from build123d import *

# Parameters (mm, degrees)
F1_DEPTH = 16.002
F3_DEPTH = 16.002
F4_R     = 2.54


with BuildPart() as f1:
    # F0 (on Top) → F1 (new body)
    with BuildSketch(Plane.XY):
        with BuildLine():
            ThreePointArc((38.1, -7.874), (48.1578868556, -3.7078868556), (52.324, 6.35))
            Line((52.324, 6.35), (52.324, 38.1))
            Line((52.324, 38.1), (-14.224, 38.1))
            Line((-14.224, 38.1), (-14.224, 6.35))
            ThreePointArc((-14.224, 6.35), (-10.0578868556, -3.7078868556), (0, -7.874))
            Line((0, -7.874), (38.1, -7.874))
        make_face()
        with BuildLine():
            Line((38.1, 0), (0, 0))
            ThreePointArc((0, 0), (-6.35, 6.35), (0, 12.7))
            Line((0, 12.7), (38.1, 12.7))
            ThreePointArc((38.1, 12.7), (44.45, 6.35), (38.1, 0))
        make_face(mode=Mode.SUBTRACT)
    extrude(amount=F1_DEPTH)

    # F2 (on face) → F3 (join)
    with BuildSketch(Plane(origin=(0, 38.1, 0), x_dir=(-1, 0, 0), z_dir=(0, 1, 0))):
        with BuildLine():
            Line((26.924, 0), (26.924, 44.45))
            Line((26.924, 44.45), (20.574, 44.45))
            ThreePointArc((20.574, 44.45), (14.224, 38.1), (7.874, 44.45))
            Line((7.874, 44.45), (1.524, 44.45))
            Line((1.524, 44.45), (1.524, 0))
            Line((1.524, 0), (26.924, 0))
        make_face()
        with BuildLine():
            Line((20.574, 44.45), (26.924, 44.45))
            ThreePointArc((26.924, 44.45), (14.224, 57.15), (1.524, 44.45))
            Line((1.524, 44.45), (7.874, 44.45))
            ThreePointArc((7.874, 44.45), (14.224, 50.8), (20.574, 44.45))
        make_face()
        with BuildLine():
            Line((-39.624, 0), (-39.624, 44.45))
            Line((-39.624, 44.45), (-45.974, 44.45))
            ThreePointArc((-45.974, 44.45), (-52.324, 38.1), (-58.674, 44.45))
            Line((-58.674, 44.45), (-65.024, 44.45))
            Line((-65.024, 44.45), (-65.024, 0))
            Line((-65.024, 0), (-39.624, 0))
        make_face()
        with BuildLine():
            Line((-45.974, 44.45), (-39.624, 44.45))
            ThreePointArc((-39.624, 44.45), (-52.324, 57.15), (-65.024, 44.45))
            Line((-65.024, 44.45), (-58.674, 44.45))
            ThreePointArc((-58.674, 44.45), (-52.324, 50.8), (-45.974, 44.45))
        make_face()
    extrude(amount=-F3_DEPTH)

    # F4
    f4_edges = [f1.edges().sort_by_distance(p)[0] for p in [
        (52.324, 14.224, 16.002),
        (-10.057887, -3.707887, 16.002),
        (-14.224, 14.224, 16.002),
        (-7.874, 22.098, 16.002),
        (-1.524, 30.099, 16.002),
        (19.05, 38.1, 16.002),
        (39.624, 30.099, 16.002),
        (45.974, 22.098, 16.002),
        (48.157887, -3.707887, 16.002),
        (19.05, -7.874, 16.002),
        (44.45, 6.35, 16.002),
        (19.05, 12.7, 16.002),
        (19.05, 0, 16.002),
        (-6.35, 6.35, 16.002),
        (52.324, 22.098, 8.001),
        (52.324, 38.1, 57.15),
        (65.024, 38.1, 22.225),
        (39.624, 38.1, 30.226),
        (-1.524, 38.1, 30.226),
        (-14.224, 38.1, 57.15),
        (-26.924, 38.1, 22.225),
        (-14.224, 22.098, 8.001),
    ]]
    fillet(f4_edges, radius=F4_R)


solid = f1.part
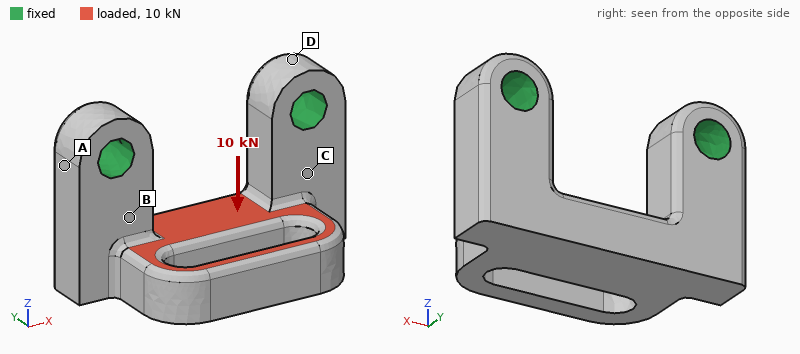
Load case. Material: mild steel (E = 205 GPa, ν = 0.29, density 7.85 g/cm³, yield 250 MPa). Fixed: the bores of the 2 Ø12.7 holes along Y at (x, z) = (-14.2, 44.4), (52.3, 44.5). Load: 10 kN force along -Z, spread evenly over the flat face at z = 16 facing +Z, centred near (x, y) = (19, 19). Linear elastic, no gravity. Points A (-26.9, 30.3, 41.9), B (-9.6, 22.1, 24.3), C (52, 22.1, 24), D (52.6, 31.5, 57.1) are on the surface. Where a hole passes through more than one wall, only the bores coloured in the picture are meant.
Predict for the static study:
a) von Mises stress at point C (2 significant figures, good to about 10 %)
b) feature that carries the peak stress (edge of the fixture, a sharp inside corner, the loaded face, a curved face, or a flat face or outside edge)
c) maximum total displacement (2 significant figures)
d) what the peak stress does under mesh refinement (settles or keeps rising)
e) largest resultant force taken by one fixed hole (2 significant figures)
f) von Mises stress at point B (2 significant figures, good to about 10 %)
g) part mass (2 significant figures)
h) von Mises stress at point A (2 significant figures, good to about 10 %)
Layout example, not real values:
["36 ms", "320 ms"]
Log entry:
["65 MPa", "a sharp inside corner", "67 µm", "keeps rising", "5.4 kN", "75 MPa", "560 g", "17 MPa"]
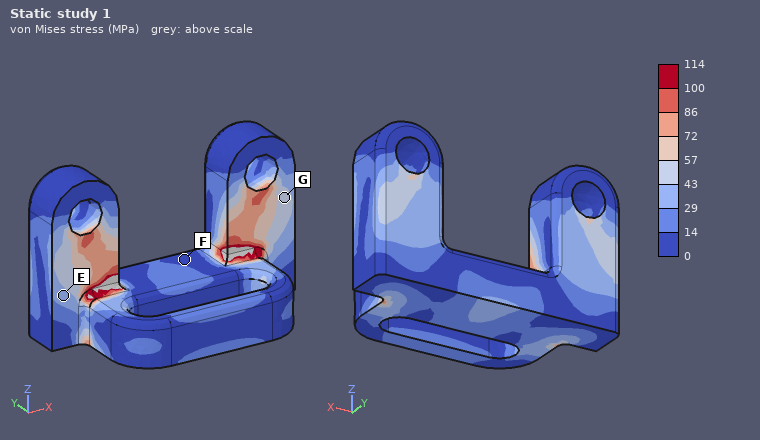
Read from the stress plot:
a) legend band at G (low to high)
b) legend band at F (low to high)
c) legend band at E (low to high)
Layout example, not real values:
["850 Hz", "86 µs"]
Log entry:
["43 to 57 MPa", "0 to 14 MPa", "29 to 43 MPa"]
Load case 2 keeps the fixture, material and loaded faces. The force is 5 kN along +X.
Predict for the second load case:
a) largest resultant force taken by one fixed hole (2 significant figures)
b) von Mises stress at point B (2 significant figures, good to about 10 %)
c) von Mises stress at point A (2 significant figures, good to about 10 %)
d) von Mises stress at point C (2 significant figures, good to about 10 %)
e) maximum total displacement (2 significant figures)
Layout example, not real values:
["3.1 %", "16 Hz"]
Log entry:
["2.6 kN", "25 MPa", "17 MPa", "24 MPa", "17 µm"]
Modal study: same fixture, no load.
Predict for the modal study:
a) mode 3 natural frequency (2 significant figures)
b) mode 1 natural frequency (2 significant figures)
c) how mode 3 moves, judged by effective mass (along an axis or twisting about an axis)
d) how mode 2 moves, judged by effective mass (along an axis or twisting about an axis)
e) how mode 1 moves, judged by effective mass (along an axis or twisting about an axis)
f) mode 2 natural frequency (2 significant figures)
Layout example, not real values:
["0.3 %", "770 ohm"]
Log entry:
["7000 Hz", "3300 Hz", "along Y", "along X", "along Y", "5500 Hz"]
